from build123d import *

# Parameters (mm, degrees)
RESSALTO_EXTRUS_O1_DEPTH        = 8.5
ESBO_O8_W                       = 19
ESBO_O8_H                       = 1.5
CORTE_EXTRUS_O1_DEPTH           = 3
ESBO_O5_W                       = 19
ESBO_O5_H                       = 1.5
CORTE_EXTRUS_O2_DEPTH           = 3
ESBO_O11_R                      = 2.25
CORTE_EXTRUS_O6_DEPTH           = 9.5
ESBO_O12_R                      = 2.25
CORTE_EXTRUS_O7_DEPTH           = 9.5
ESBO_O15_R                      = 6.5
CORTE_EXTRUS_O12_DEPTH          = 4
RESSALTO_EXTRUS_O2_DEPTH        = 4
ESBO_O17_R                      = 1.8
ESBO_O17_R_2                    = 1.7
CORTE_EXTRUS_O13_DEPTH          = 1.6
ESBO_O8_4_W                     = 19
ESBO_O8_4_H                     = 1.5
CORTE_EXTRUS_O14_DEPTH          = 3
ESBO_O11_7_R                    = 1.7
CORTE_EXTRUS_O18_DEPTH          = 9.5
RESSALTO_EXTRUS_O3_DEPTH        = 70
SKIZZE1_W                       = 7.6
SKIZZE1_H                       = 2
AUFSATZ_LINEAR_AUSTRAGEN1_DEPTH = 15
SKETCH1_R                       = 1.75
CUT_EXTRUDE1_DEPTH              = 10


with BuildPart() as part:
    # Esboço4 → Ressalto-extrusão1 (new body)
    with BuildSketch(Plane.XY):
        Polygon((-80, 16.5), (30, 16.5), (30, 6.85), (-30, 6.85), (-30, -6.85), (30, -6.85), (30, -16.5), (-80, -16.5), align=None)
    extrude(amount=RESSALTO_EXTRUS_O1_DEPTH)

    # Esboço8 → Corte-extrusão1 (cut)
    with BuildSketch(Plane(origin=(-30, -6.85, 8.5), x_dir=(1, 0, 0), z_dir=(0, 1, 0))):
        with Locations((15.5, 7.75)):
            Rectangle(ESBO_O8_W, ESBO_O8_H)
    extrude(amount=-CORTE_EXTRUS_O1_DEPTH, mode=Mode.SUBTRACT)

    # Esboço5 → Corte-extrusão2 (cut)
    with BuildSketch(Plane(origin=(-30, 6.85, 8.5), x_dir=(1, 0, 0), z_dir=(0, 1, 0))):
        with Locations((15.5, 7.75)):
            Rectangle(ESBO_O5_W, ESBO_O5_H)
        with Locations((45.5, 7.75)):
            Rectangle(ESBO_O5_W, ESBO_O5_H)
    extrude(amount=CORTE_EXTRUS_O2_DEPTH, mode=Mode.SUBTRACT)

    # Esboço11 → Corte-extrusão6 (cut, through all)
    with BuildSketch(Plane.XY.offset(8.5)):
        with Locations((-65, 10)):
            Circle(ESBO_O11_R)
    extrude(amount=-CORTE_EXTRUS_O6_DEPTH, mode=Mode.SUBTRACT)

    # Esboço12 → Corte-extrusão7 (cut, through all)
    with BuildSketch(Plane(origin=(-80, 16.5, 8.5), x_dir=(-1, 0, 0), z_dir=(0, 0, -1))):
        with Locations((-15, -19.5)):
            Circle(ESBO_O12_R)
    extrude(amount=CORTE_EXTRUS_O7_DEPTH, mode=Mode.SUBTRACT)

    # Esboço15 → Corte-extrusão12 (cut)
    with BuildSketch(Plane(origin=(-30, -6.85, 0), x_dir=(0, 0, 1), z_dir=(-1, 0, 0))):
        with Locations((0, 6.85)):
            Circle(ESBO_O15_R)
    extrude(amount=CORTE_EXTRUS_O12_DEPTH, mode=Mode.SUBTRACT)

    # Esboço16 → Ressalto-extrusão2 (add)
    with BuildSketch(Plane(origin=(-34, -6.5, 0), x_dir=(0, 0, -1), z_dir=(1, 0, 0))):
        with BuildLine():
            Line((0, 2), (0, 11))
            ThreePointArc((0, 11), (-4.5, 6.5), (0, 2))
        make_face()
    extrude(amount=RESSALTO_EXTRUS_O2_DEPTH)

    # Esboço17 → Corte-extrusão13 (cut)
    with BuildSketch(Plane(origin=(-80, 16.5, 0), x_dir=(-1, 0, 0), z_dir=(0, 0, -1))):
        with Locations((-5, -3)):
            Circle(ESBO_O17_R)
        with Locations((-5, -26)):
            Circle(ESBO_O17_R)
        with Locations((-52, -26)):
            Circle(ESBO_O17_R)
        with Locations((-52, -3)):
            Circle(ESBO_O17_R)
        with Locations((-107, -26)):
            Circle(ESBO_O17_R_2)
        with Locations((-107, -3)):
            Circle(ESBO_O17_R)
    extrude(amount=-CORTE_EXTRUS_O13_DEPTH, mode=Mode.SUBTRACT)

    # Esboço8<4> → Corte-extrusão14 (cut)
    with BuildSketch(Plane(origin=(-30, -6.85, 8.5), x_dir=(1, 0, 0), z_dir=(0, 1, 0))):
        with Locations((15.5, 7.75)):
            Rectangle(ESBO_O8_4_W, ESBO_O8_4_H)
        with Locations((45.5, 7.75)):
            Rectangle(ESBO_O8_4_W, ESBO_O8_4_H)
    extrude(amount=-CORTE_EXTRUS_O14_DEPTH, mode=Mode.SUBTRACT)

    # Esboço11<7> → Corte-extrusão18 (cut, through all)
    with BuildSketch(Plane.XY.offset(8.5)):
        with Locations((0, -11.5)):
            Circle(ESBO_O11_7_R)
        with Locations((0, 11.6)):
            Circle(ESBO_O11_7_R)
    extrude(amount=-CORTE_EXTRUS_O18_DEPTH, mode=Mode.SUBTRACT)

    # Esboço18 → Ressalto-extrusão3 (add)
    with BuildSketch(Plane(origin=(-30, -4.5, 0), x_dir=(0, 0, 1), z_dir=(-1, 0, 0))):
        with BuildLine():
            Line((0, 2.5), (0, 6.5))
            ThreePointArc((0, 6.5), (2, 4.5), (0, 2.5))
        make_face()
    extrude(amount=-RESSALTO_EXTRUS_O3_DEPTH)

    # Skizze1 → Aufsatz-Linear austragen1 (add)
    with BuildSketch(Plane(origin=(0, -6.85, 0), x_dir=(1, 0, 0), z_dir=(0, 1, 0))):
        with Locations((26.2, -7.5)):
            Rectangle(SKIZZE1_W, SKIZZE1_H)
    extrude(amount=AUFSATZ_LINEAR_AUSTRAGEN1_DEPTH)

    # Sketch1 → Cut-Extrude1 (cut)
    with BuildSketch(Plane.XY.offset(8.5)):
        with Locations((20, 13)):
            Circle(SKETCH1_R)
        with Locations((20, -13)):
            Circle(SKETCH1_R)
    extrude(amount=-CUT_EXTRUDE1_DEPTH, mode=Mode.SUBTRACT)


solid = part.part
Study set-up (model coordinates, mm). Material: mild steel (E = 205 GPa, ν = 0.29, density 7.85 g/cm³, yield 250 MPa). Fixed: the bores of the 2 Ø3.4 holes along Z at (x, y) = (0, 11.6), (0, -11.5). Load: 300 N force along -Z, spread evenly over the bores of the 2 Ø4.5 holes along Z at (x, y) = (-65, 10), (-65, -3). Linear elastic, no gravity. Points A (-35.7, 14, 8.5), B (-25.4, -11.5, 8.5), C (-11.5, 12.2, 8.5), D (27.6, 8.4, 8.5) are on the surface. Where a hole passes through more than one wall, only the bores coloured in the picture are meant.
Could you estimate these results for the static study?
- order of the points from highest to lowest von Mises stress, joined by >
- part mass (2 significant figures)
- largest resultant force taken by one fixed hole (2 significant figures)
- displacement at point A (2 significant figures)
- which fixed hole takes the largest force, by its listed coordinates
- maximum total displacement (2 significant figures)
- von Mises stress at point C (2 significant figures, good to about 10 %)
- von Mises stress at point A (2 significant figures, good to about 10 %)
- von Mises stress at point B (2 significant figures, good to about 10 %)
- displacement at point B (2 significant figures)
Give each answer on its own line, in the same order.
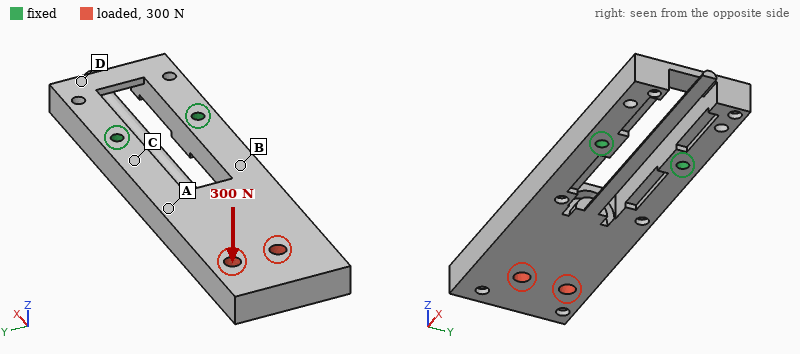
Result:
C > B > A > D
180 g
170 N
0.059 mm
(0, 11.6)
0.20 mm
77 MPa
29 MPa
56 MPa
0.030 mm
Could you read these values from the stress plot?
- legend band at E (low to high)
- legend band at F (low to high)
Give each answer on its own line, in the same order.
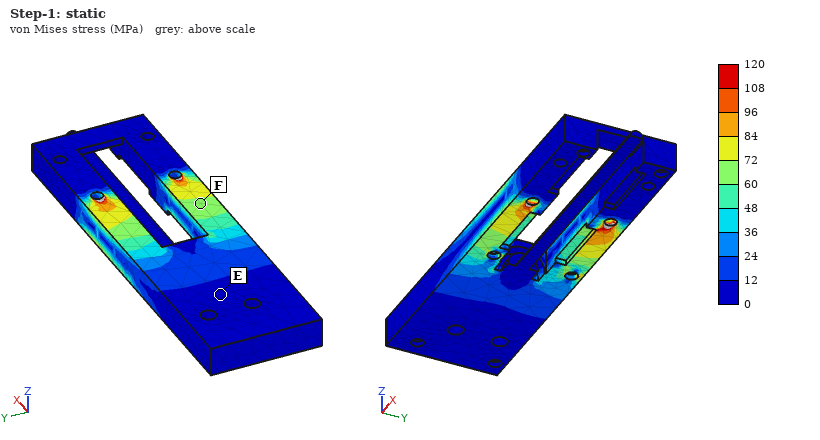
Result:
0 to 12 MPa
60 to 72 MPa
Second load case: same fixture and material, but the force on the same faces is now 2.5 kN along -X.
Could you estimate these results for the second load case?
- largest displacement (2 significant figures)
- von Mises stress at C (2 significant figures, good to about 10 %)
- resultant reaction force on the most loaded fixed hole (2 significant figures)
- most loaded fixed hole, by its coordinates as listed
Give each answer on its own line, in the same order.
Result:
10 µm
18 MPa
1.6 kN
(0, 11.6)
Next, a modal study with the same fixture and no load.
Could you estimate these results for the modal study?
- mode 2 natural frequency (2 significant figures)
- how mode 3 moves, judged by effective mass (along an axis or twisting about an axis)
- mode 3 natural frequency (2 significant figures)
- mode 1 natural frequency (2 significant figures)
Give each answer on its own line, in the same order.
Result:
560 Hz
along Z
830 Hz
300 Hz
